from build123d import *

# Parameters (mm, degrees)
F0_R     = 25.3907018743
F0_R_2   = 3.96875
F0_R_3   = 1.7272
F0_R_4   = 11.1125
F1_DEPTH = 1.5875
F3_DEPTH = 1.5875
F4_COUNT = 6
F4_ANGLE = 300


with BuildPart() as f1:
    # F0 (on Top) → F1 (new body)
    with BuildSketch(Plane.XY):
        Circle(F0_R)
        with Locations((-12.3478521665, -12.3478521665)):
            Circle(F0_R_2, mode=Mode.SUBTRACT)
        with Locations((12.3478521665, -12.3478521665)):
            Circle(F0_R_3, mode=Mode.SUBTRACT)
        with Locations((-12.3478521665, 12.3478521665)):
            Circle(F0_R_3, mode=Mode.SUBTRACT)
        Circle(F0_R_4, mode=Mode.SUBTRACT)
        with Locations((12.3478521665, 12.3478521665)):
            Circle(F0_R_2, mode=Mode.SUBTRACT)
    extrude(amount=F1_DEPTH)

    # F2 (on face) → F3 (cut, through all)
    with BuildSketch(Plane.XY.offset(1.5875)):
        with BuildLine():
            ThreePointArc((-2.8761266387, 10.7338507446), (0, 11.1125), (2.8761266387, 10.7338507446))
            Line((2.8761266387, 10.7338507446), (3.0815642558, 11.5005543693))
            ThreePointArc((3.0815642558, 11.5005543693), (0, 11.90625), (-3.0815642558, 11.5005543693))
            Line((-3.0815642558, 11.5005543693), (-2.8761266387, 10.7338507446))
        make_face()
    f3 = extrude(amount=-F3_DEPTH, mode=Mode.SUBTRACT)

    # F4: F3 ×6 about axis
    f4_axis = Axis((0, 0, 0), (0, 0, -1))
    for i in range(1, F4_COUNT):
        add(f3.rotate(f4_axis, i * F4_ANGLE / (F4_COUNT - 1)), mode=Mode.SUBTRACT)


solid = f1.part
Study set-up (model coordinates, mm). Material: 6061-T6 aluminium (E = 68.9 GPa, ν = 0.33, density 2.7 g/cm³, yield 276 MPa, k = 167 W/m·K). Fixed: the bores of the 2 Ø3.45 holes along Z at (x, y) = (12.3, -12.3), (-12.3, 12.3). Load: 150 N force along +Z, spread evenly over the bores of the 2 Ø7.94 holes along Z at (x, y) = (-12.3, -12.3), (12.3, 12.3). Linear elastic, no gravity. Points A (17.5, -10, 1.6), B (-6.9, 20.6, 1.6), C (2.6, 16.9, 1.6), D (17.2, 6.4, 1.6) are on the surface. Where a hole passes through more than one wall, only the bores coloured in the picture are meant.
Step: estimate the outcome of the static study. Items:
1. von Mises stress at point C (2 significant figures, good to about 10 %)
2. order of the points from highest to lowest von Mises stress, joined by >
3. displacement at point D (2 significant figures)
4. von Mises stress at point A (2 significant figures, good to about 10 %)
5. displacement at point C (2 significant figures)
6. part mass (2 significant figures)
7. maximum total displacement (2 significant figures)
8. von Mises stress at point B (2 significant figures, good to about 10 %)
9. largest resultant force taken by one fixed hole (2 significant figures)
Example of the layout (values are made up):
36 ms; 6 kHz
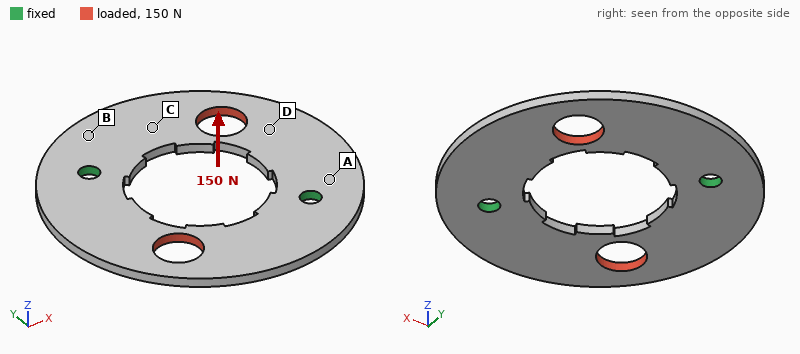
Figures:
26 MPa; A > B > C > D; 0.25 mm; 84 MPa; 0.18 mm; 6.4 g; 0.45 mm; 63 MPa; 75 N
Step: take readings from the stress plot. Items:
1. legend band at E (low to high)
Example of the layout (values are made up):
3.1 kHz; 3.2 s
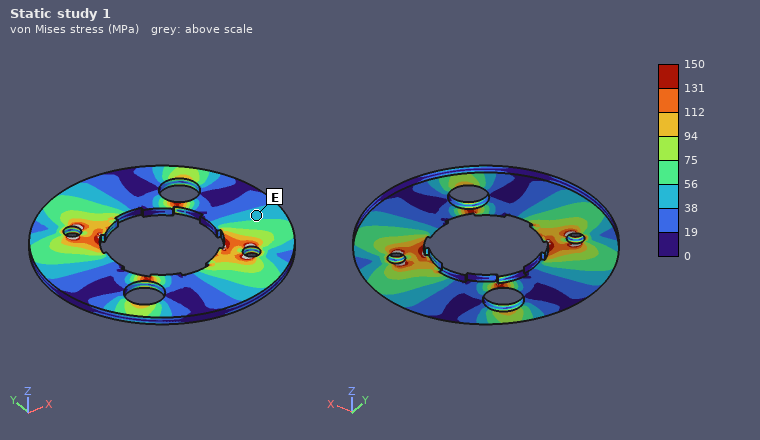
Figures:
38 to 56 MPa
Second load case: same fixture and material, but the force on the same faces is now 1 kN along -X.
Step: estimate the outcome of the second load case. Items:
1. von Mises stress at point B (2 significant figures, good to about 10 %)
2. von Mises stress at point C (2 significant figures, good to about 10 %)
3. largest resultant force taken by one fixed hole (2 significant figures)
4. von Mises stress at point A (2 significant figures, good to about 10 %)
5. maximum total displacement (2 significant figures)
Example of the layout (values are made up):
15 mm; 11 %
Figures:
14 MPa; 18 MPa; 500 N; 13 MPa; 16 µm
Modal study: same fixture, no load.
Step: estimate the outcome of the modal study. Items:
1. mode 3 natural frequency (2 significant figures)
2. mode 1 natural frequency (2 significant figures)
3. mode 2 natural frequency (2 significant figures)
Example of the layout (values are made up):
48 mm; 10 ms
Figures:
4900 Hz; 2100 Hz; 2100 Hz
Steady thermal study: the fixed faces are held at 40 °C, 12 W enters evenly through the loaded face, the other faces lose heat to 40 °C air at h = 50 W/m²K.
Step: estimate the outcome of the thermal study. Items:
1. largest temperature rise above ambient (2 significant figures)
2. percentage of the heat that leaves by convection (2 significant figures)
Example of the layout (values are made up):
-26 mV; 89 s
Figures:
21 K; 14 %
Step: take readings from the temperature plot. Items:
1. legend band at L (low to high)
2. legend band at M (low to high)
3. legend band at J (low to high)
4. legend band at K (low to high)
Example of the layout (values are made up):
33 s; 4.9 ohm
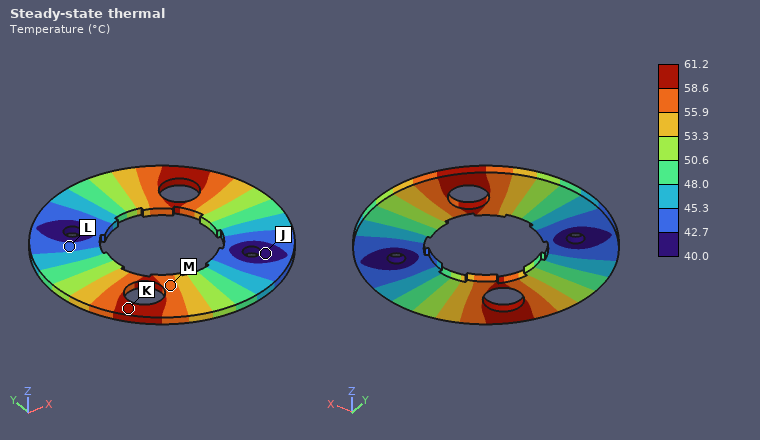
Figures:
42.7 to 45.3 °C; 55.9 to 58.6 °C; 40.0 to 42.7 °C; 58.6 to 61.2 °C
